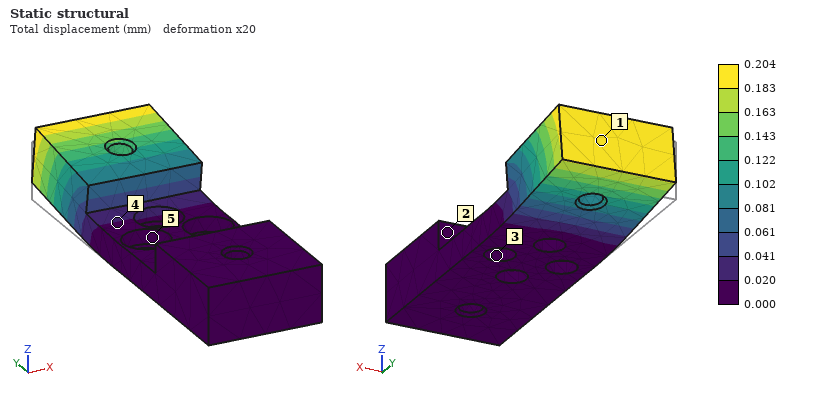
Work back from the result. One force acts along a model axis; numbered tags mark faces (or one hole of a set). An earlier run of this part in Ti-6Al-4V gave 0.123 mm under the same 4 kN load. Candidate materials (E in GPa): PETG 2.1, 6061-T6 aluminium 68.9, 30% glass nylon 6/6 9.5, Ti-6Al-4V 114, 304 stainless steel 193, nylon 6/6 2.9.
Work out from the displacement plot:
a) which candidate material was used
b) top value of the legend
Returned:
6061-T6 aluminium
0.204 mm
